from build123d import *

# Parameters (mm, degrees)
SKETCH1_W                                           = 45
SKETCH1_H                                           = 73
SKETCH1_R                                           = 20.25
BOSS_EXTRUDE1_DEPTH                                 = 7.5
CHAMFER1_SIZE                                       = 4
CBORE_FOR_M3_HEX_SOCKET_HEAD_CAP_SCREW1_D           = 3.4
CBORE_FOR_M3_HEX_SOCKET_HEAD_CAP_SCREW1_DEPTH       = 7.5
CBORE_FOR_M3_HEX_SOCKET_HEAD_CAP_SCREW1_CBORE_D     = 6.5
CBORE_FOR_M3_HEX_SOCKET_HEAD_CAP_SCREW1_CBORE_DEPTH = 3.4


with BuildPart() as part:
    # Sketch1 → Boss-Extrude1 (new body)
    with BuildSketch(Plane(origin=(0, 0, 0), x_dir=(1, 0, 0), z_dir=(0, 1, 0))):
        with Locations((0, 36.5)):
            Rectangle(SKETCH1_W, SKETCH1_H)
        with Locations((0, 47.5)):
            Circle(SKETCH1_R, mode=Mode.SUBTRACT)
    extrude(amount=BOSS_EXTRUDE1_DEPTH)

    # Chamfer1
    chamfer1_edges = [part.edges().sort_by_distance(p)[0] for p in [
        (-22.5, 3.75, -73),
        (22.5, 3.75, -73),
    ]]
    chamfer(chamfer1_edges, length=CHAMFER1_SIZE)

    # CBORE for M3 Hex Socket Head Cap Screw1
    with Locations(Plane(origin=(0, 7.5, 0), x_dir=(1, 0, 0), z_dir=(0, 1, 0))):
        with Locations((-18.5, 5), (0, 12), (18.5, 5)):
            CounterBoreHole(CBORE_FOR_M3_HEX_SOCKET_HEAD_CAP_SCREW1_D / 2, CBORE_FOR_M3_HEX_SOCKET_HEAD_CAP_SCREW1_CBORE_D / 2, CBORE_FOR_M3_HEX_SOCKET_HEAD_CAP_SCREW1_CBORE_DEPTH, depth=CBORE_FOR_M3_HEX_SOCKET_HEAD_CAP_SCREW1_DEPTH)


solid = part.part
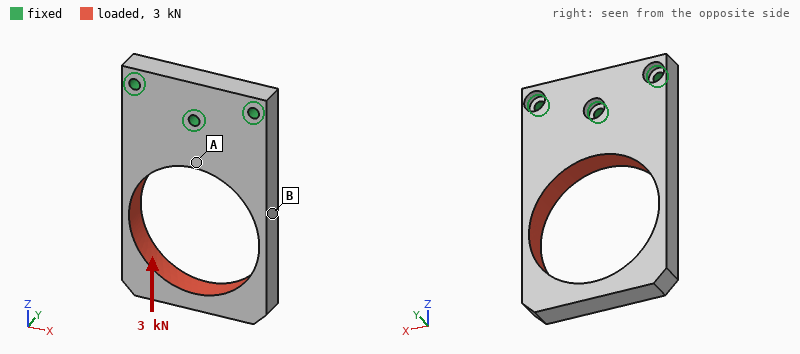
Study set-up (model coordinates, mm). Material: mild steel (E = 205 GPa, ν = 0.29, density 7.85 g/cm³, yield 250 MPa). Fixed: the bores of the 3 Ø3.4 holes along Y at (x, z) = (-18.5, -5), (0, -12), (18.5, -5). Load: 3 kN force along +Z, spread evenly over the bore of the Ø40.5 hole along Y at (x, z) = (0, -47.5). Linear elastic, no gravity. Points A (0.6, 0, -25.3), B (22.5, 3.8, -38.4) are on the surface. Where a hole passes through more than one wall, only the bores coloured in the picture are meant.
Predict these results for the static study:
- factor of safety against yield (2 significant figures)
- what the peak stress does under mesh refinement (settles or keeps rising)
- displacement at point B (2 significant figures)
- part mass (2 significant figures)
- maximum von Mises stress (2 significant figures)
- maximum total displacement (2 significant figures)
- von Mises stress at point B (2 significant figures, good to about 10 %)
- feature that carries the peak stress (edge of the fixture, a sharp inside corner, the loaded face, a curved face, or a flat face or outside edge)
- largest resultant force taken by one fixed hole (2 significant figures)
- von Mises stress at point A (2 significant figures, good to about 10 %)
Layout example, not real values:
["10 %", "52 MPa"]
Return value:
["1.9", "settles", "11 µm", "110 g", "130 MPa", "34 µm", "82 MPa", "the loaded face", "1.1 kN", "19 MPa"]
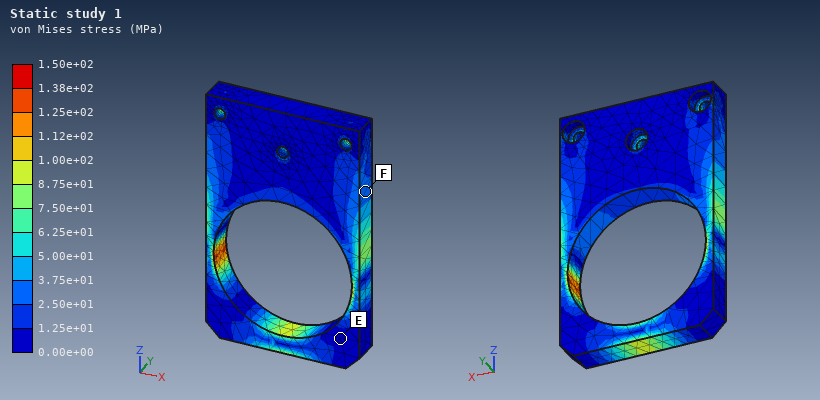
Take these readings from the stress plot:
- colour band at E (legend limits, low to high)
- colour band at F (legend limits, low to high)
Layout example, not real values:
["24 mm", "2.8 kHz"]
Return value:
["0.00e+00 to 1.25e+01 MPa", "2.50e+01 to 3.75e+01 MPa"]
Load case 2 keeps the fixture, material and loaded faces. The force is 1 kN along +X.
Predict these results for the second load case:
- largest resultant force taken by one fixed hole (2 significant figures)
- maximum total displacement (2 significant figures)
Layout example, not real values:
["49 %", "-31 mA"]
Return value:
["950 N", "74 µm"]
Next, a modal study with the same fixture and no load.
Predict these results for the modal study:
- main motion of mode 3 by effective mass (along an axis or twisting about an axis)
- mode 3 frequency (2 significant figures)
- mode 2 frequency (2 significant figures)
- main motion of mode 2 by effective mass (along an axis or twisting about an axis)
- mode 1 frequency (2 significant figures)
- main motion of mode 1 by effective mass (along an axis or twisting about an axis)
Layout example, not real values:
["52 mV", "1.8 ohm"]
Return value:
["twisting about Z", "2900 Hz", "2600 Hz", "along X", "1200 Hz", "along Y"]
